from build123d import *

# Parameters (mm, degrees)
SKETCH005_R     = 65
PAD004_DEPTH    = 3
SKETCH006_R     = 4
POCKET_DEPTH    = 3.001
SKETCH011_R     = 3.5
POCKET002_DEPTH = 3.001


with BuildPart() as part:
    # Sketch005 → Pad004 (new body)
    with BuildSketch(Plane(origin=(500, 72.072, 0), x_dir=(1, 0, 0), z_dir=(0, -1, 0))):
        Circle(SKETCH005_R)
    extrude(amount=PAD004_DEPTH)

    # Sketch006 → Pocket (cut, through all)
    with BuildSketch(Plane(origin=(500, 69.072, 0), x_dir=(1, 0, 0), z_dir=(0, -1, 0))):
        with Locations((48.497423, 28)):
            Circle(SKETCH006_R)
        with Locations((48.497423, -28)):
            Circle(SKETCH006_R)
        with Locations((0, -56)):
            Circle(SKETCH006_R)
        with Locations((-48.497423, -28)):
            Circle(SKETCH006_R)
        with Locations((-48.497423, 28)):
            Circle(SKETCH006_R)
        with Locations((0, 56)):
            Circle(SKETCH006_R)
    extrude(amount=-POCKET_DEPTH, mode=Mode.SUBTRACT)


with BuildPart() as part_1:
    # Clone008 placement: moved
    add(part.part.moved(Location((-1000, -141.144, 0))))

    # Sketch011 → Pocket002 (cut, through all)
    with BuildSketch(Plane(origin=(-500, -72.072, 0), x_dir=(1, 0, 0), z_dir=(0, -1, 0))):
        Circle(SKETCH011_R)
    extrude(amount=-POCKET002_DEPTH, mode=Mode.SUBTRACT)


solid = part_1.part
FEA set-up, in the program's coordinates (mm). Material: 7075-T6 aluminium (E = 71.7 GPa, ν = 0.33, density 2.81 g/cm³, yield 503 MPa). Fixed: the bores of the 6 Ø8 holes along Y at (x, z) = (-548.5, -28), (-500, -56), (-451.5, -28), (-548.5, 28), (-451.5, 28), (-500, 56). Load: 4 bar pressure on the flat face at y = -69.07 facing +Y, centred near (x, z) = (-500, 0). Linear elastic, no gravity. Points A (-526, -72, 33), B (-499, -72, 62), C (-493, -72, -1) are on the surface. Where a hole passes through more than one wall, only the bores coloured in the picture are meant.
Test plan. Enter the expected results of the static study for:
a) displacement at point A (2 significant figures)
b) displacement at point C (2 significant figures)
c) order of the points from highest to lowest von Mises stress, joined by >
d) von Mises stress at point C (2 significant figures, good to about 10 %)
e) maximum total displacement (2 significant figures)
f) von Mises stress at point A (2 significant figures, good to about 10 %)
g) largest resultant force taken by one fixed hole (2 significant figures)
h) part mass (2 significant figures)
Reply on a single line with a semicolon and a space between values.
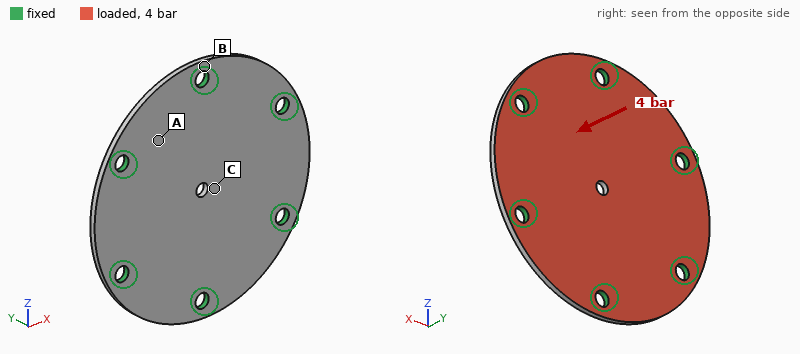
0.11 mm; 0.37 mm; C > A > B; 70 MPa; 0.39 mm; 51 MPa; 860 N; 110 g
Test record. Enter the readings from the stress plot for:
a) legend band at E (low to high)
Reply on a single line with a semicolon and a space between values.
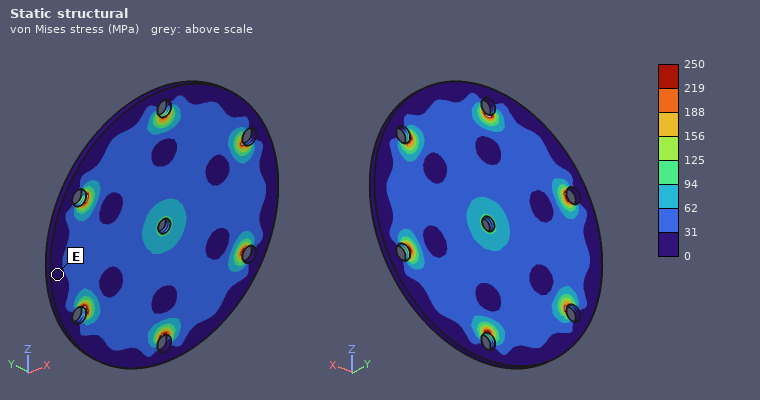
0 to 31 MPa
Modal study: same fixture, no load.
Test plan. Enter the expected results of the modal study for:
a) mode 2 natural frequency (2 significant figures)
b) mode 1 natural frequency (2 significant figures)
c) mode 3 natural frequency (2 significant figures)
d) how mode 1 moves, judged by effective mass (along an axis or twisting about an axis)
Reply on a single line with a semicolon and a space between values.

4500 Hz; 2200 Hz; 4500 Hz; along Y
